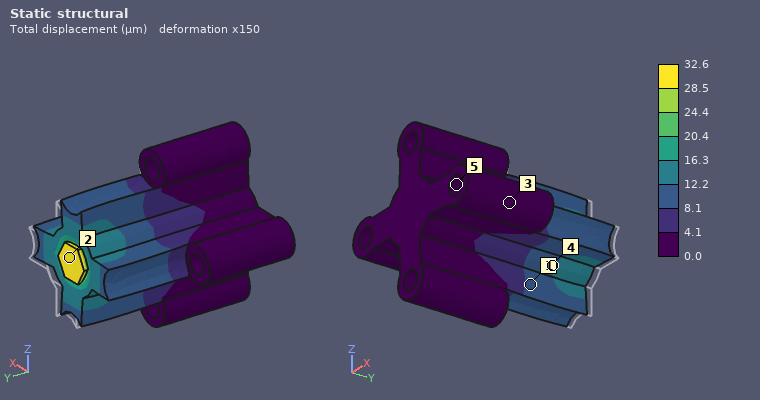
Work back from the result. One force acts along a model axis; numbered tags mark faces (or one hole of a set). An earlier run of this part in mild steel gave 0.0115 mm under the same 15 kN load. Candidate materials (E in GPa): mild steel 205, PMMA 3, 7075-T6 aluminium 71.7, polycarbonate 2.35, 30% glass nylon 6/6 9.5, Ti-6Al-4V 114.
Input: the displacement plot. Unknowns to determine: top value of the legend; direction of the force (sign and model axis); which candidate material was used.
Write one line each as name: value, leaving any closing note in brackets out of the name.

top value of the legend: 32.6 µm
direction of the force: -Y
which candidate material was used: 7075-T6 aluminium
